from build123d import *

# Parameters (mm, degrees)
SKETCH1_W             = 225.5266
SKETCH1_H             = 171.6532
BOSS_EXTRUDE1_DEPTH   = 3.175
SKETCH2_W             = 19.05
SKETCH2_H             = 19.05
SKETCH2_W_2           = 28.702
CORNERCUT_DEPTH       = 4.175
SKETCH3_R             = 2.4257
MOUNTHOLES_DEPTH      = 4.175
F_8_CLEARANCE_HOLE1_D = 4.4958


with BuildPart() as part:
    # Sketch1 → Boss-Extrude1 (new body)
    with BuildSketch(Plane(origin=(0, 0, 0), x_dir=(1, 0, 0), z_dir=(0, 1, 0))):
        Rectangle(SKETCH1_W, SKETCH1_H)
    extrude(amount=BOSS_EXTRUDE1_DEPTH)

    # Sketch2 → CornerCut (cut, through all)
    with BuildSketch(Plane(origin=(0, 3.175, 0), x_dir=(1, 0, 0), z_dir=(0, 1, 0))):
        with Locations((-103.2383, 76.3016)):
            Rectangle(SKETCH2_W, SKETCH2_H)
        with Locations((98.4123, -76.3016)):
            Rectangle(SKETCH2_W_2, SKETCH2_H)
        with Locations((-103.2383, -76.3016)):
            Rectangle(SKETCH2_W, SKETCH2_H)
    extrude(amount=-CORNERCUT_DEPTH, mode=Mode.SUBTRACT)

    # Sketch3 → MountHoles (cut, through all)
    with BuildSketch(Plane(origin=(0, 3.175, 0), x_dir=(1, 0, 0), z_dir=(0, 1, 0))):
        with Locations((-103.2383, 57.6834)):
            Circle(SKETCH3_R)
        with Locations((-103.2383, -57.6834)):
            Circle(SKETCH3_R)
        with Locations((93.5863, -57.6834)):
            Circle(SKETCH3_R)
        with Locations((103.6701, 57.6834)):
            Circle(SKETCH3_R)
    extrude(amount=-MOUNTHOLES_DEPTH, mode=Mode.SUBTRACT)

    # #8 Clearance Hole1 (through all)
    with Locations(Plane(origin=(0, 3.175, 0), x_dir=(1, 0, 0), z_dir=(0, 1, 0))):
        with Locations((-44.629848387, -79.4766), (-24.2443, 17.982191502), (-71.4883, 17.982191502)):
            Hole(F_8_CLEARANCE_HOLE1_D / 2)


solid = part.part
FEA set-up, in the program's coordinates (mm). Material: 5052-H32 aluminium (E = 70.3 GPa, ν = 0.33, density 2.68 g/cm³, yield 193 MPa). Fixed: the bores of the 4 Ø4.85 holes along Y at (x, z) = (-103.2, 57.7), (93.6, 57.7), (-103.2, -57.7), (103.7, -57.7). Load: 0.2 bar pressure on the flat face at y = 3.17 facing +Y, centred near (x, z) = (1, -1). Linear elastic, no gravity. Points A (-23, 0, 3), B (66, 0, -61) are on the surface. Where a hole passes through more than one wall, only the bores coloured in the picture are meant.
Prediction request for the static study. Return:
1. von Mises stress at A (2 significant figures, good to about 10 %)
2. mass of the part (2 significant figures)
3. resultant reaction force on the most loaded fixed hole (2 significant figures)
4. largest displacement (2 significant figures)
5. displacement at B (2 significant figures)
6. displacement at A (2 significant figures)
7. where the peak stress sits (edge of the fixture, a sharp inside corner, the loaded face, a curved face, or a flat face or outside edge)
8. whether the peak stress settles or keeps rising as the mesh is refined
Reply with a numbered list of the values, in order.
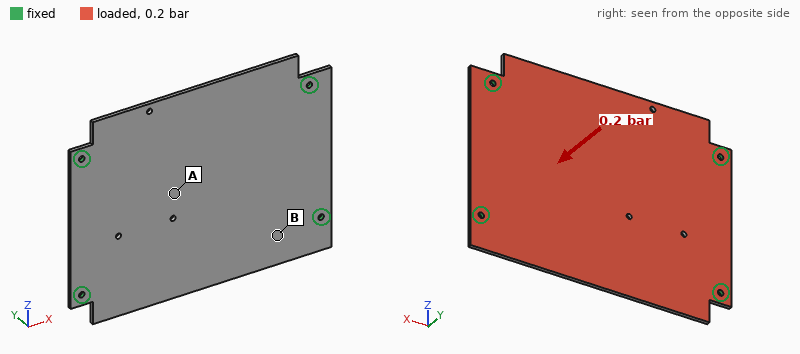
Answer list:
1. 20 MPa
2. 320 g
3. 200 N
4. 0.75 mm
5. 0.29 mm
6. 0.65 mm
7. edge of the fixture
8. keeps rising
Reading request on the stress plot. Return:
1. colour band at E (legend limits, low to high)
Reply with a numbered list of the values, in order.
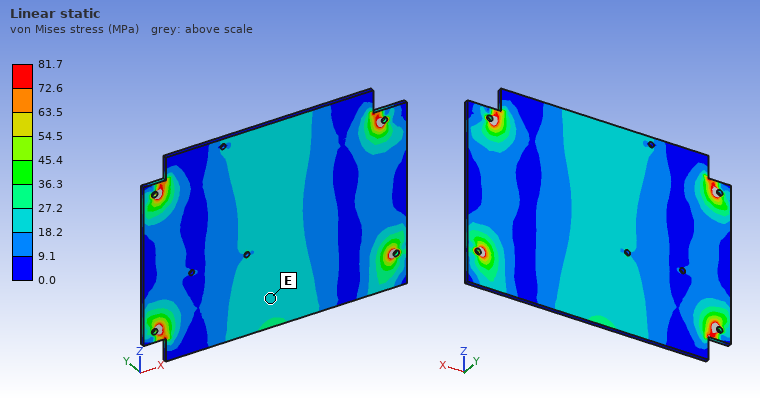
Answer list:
1. 18.2 to 27.2 MPa
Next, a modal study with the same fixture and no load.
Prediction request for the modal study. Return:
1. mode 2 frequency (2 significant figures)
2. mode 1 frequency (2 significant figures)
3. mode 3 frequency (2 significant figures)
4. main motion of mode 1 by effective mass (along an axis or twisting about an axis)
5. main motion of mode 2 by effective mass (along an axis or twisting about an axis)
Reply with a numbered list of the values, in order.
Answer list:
1. 460 Hz
2. 330 Hz
3. 800 Hz
4. along Y
5. twisting about X
